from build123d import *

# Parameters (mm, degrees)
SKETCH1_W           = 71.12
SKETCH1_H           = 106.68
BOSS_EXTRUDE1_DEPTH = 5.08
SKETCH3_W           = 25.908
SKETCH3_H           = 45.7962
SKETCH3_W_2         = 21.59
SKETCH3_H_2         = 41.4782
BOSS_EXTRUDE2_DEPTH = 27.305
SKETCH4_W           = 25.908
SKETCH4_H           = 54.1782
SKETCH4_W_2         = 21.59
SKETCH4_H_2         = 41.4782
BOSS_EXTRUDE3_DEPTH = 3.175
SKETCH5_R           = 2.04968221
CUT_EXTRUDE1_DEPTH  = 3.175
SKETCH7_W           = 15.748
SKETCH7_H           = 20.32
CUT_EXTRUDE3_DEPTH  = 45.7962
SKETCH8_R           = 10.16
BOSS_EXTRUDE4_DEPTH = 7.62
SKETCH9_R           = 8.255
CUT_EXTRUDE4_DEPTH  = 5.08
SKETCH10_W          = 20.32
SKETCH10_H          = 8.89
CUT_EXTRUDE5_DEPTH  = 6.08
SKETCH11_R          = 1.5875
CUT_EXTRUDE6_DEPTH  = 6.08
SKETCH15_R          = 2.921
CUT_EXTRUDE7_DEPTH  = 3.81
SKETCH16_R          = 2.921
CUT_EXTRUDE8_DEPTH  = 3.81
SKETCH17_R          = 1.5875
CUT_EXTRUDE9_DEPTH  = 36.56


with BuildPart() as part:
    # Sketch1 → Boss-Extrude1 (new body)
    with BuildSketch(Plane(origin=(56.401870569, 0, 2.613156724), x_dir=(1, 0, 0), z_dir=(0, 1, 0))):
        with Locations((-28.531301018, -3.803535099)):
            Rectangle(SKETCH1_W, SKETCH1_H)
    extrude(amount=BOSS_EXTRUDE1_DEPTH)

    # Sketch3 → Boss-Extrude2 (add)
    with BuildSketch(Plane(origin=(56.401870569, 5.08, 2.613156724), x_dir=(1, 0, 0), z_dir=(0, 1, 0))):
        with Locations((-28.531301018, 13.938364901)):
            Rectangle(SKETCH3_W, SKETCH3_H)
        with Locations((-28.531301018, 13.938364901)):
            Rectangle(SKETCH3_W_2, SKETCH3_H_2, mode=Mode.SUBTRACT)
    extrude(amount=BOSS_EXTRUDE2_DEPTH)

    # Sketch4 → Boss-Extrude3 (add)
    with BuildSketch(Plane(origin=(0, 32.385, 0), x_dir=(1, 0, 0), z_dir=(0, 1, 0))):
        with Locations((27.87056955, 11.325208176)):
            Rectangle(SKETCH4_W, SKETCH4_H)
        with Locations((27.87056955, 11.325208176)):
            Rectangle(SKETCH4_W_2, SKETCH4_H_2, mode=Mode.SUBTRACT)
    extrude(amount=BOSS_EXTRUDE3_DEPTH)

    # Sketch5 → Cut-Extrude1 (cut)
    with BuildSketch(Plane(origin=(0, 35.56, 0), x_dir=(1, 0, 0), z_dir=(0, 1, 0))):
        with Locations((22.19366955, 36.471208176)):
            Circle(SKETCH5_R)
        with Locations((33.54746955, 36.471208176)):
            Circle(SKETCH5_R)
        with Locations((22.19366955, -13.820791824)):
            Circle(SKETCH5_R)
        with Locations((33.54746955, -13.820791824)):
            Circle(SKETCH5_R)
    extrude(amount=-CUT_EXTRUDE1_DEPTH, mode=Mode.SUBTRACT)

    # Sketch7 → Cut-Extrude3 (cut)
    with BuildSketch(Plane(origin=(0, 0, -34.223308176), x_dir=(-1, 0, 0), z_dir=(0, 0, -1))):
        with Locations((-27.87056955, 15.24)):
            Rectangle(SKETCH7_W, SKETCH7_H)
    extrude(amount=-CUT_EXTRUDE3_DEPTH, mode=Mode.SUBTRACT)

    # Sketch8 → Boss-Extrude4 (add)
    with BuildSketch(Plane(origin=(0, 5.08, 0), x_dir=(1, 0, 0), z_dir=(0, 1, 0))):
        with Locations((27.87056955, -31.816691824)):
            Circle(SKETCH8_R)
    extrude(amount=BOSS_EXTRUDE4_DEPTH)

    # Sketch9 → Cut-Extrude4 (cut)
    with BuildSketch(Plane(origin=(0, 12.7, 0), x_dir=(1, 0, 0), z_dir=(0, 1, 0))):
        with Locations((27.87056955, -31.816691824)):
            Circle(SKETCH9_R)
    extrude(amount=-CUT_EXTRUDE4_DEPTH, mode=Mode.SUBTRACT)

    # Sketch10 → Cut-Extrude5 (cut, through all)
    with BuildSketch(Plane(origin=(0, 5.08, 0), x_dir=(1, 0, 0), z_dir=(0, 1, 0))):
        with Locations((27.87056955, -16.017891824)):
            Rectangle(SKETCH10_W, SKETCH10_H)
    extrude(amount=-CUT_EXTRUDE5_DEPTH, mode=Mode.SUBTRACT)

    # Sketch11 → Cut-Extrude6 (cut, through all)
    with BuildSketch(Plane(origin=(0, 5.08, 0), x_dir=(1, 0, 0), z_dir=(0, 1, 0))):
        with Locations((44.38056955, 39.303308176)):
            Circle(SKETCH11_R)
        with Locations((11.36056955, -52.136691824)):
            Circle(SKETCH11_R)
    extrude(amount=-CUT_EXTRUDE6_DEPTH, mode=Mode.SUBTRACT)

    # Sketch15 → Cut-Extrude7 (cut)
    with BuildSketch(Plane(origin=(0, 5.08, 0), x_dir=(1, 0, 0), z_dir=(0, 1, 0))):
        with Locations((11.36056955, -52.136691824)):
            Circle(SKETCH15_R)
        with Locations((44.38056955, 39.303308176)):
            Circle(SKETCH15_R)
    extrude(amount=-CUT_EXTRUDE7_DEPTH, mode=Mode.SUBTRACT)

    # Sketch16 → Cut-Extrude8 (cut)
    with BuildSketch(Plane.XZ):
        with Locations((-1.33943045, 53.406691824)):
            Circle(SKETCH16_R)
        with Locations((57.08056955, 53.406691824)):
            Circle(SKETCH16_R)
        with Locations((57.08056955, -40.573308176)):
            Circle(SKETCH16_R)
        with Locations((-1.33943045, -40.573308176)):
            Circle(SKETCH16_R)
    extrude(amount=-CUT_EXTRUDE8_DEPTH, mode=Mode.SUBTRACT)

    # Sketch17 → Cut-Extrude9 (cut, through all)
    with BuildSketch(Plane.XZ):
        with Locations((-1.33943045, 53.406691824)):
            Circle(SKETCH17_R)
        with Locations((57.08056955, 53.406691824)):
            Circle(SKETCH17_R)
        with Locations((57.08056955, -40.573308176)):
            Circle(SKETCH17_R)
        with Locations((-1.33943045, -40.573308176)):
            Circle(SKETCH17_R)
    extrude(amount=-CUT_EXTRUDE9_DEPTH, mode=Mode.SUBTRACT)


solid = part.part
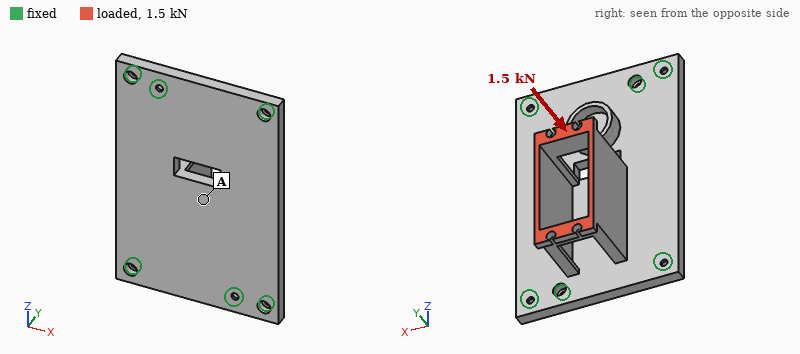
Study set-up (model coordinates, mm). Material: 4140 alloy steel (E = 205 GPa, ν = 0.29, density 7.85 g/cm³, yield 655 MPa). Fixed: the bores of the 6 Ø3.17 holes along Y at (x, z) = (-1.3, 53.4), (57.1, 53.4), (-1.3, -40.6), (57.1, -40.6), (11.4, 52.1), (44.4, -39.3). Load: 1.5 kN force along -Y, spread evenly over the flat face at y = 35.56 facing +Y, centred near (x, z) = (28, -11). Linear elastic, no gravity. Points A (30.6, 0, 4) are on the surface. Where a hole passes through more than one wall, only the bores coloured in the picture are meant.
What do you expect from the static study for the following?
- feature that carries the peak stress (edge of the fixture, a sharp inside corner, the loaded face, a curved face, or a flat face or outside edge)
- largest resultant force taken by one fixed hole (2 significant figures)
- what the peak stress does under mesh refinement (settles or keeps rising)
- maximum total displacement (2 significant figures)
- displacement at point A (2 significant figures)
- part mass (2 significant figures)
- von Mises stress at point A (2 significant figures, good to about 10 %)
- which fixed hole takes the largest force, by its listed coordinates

edge of the fixture
1.3 kN
keeps rising
65 µm
44 µm
360 g
16 MPa
(44.4, -39.3)
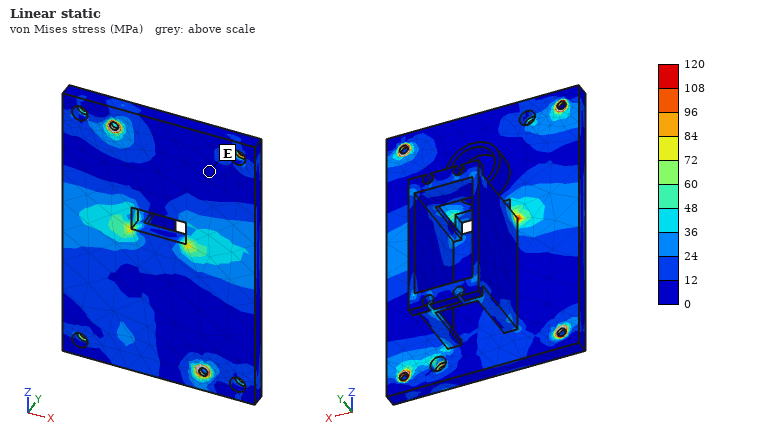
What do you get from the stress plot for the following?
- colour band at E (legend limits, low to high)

0 to 12 MPa
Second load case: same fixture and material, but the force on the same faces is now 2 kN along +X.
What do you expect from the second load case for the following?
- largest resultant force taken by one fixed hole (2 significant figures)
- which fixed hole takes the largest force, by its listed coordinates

1.2 kN
(57.1, -40.6)
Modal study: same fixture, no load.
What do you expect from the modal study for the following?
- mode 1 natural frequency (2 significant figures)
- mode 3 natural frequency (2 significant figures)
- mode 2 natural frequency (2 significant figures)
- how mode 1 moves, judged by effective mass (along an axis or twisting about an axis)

1900 Hz
4400 Hz
2700 Hz
along Y
